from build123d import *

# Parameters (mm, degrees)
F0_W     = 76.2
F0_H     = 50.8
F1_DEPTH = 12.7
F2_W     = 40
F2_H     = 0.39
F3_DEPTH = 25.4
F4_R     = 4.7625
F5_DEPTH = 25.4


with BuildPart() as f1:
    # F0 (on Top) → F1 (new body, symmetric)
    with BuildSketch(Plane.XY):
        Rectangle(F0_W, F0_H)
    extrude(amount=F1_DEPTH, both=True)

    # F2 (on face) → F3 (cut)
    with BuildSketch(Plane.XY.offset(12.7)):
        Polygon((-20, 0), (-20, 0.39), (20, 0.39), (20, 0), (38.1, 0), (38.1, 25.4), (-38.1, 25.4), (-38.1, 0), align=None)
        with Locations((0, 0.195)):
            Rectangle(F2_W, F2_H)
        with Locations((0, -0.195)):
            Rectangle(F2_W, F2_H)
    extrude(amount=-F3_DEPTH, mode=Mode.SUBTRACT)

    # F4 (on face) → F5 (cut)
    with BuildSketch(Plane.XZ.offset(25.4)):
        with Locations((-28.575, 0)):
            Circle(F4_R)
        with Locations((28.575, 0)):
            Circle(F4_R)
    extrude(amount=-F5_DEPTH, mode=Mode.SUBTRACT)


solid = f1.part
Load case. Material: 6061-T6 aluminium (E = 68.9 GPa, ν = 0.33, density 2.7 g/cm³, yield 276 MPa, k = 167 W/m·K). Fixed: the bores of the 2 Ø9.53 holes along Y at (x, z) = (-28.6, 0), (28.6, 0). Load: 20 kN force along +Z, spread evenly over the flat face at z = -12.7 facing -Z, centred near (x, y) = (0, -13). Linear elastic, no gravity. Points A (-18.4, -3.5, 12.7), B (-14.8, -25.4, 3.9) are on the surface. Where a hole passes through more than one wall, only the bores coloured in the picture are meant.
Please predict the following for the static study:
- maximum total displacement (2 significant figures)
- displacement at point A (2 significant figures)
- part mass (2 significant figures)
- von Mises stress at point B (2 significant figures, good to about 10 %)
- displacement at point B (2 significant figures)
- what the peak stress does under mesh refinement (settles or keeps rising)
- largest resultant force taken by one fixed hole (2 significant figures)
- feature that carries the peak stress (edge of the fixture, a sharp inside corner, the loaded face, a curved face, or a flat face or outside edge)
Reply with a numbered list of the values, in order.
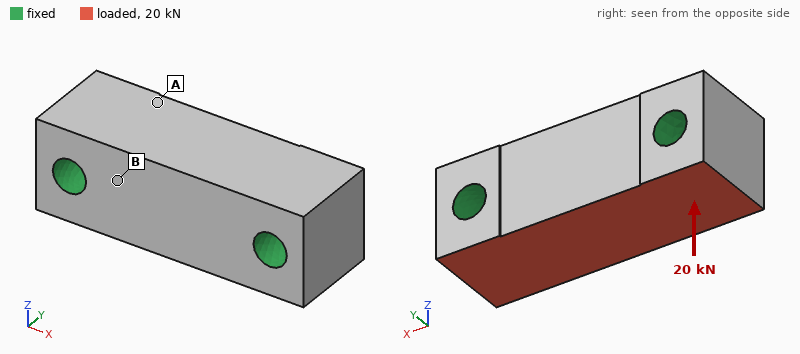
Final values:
1. 12 µm
2. 5.4 µm
3. 120 g
4. 16 MPa
5. 6.5 µm
6. keeps rising
7. 10 kN
8. edge of the fixture
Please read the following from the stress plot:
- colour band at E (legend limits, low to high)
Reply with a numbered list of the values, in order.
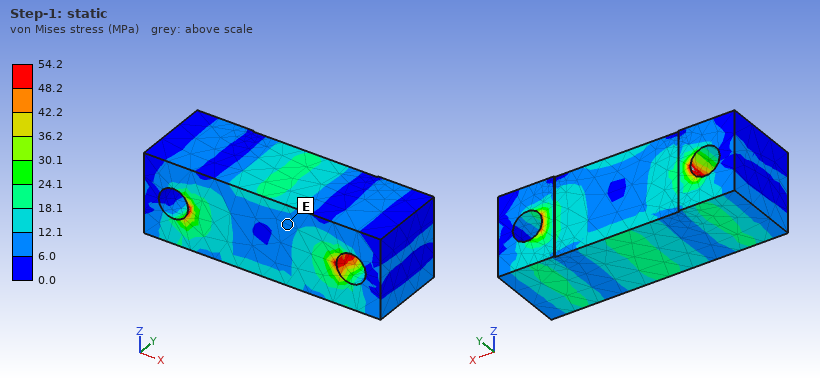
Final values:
1. 6.0 to 12.1 MPa
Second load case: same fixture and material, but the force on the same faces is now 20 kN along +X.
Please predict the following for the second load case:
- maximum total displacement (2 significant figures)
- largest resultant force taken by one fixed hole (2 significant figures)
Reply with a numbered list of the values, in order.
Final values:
1. 9.2 µm
2. 11 kN
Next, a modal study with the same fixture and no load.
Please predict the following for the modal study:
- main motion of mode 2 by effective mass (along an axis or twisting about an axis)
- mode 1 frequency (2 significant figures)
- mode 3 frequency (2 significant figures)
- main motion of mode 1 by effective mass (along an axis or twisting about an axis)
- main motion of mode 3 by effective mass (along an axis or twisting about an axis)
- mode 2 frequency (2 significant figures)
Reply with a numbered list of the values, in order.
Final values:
1. along Y
2. 21 kHz
3. 27 kHz
4. along Z
5. twisting about X
6. 23 kHz
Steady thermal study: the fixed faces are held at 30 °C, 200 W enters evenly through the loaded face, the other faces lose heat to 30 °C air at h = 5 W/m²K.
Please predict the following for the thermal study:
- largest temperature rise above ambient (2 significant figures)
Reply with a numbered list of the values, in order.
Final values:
1. 15 K
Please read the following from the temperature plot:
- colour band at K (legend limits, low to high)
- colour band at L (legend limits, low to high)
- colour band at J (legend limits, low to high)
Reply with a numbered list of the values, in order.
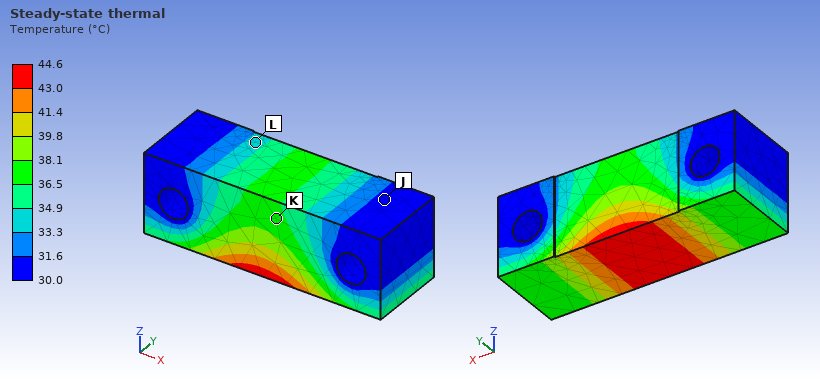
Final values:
1. 36.5 to 38.1 °C
2. 33.3 to 34.9 °C
3. 30.0 to 31.6 °C
